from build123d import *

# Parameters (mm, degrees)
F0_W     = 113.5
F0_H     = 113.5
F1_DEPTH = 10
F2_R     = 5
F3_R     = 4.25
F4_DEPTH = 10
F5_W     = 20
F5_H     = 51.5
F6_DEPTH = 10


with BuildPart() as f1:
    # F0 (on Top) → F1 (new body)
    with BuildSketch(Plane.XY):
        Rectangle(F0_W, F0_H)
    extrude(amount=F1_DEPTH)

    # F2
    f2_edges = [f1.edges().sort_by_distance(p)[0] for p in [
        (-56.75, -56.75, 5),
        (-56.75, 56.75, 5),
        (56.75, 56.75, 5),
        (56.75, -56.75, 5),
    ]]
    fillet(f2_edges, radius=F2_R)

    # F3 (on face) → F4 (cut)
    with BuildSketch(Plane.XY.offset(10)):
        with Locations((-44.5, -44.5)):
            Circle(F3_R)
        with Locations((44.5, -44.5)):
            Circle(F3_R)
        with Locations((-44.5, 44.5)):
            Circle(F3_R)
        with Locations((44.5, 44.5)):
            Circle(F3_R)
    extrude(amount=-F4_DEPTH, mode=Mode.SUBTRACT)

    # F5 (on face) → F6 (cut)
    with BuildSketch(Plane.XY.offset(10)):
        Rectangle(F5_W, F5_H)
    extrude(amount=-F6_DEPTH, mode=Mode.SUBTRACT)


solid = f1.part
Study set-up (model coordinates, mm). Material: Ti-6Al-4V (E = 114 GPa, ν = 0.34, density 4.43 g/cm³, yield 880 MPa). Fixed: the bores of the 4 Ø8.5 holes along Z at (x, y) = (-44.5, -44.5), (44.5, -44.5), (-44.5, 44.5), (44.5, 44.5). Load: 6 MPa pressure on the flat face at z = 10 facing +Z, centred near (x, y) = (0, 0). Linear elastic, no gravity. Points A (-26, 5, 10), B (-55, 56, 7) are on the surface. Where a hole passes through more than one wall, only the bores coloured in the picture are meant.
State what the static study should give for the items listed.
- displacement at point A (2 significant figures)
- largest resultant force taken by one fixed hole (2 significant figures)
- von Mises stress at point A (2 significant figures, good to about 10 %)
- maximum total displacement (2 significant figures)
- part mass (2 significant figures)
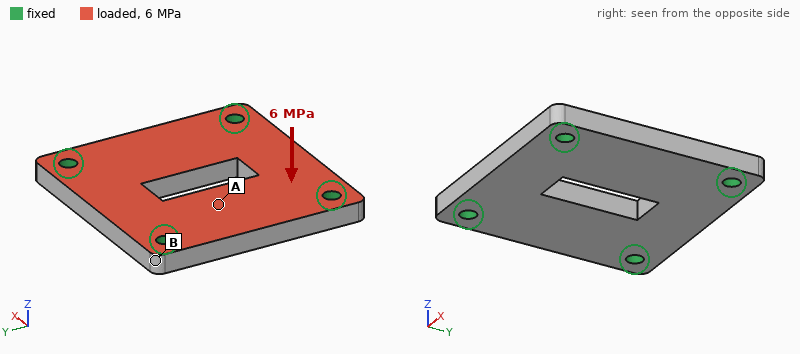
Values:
0.21 mm
17 kN
120 MPa
0.31 mm
510 g
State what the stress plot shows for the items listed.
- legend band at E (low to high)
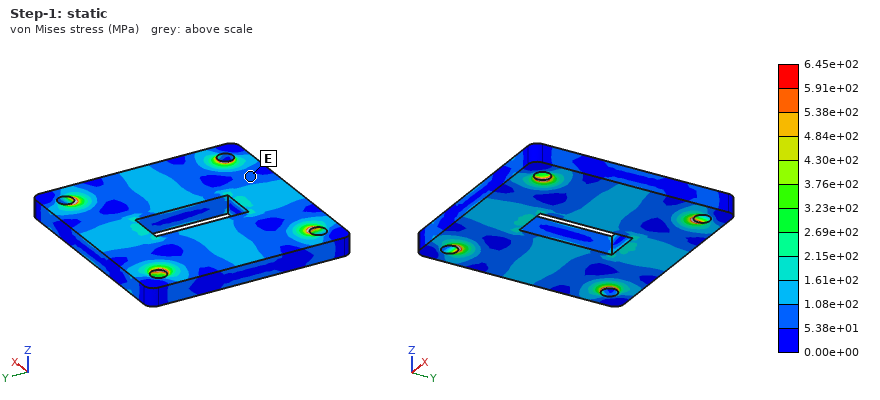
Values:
5.38e+01 to 1.08e+02 MPa
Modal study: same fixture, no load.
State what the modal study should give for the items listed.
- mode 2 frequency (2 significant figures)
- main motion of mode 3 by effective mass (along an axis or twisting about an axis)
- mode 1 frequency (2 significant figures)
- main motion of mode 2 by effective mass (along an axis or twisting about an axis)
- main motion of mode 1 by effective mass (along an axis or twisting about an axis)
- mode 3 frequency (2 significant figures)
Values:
6300 Hz
twisting about X
4400 Hz
twisting about Y
along Z
6900 Hz
